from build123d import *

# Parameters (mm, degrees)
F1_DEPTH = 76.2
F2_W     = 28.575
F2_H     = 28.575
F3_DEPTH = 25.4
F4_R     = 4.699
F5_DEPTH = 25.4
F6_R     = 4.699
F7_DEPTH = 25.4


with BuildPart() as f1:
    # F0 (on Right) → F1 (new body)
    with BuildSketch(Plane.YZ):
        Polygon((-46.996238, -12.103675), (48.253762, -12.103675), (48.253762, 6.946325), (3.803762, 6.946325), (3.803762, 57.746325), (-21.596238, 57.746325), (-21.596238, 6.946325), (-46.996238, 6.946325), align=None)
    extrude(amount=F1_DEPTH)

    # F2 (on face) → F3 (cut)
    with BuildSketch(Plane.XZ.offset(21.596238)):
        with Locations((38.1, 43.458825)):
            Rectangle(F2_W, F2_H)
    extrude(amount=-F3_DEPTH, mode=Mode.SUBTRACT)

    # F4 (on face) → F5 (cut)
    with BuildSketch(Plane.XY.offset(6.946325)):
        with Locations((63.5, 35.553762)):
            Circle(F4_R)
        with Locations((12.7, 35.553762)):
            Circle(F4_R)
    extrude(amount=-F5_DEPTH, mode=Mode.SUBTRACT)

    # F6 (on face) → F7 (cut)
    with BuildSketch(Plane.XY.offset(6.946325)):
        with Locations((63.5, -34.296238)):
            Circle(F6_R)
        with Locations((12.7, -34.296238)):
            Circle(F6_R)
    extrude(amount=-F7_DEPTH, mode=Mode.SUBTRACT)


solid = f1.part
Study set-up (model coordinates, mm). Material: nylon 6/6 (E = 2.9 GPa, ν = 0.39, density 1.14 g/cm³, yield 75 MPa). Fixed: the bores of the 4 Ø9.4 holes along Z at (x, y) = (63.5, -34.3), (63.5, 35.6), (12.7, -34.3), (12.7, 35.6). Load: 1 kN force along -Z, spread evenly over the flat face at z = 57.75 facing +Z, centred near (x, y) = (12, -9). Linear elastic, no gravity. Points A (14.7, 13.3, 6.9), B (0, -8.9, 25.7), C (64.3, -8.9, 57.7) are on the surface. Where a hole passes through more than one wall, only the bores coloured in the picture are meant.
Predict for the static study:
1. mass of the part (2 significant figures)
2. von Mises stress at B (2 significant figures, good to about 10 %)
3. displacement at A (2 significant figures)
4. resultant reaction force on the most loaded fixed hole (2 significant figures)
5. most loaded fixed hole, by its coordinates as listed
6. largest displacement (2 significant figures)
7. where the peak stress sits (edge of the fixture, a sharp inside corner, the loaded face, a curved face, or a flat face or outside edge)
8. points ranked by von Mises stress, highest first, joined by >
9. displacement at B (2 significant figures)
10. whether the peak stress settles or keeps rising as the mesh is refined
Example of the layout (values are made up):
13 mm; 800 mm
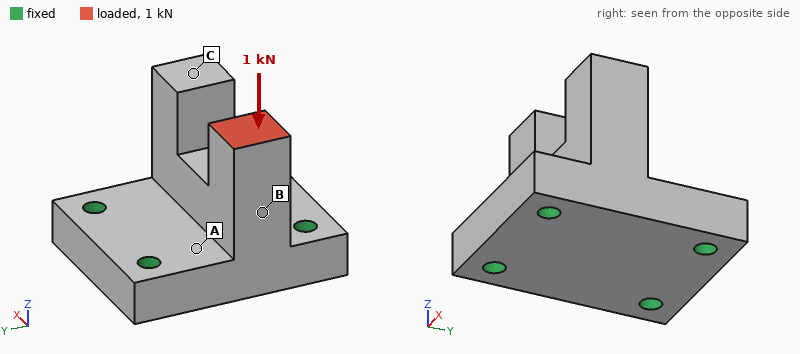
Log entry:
240 g; 1.8 MPa; 23 µm; 660 N; (12.7, -34.3); 98 µm; edge of the fixture; B > A > C; 59 µm; keeps rising
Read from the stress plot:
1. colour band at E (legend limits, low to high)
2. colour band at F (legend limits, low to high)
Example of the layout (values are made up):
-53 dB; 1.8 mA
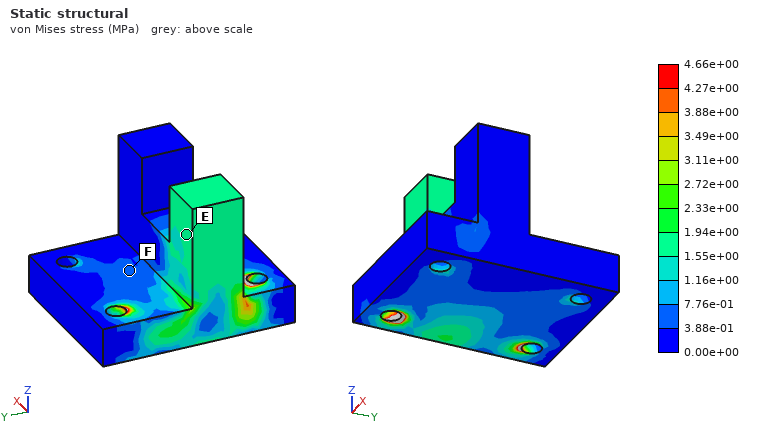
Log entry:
1.55e+00 to 1.94e+00 MPa; 3.88e-01 to 7.76e-01 MPa
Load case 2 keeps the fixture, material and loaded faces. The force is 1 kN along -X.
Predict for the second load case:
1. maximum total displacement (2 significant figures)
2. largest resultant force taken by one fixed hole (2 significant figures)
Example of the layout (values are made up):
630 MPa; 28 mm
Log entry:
0.49 mm; 880 N
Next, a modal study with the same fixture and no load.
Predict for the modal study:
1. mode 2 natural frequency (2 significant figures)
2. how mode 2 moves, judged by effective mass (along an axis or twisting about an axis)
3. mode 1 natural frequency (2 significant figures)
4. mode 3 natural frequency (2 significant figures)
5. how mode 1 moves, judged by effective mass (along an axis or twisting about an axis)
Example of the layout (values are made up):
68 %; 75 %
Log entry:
1900 Hz; along X; 1800 Hz; 2100 Hz; along Y
